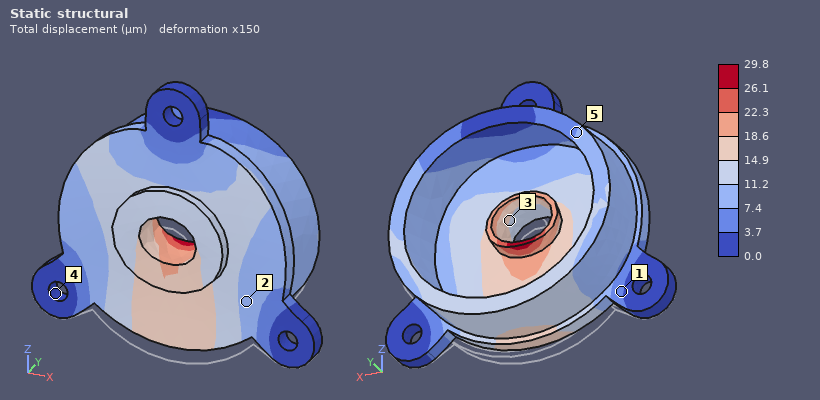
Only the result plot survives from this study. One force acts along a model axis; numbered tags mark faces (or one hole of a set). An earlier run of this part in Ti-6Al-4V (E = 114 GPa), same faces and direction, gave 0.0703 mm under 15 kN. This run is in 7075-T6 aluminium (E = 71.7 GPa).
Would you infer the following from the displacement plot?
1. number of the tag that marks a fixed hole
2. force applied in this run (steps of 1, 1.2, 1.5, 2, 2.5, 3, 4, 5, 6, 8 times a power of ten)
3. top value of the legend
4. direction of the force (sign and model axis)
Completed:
4
4 kN
29.8 µm
+Z
